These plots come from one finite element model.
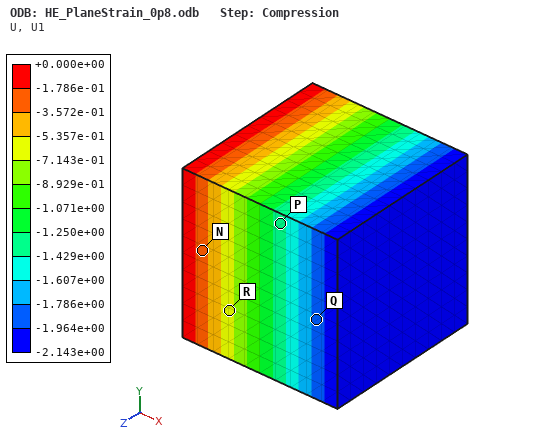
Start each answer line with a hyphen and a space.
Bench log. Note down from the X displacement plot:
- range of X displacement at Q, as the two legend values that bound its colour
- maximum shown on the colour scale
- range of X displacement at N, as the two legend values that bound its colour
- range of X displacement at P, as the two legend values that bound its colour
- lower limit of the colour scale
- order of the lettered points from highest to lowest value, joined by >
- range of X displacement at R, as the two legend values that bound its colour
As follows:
- -1.964e+00 to -1.786e+00
- +0.000e+00
- -3.572e-01 to -1.786e-01
- -1.429e+00 to -1.250e+00
- -2.143e+00
- N > R > P > Q
- -7.143e-01 to -5.357e-01
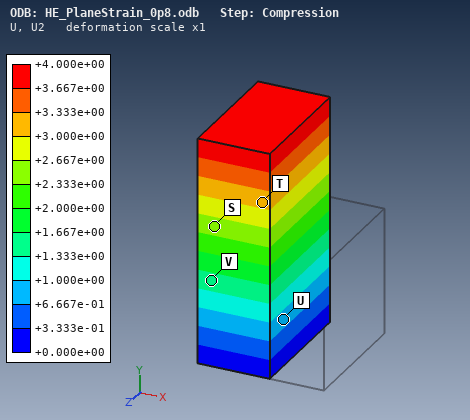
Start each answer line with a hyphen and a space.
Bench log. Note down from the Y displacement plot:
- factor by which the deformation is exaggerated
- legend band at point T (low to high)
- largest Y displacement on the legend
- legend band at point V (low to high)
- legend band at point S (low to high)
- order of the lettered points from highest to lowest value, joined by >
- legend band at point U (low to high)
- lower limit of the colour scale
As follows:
- 1
- +3.000e+00 to +3.333e+00
- +4.000e+00
- +1.333e+00 to +1.667e+00
- +2.333e+00 to +2.667e+00
- T > S > V > U
- +6.667e-01 to +1.000e+00
- +0.000e+00
